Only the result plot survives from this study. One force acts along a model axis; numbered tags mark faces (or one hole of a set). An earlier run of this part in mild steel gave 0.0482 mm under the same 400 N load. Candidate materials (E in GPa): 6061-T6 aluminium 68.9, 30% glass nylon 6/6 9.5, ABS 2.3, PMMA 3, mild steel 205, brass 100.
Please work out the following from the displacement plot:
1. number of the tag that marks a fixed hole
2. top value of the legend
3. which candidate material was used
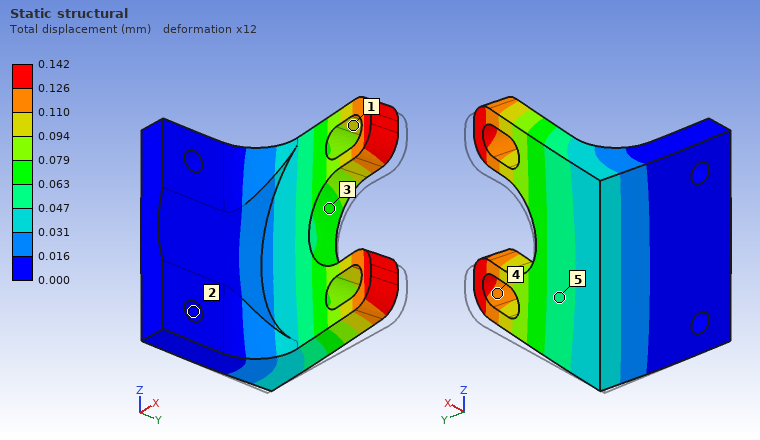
2
0.142 mm
6061-T6 aluminium
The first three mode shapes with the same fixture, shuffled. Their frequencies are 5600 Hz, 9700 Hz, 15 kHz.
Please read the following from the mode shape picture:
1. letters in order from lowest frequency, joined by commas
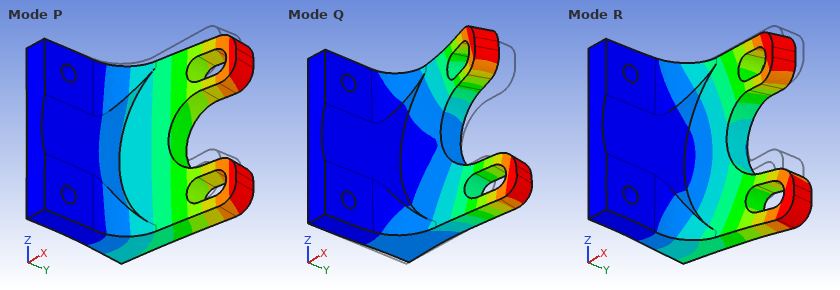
P, R, Q
